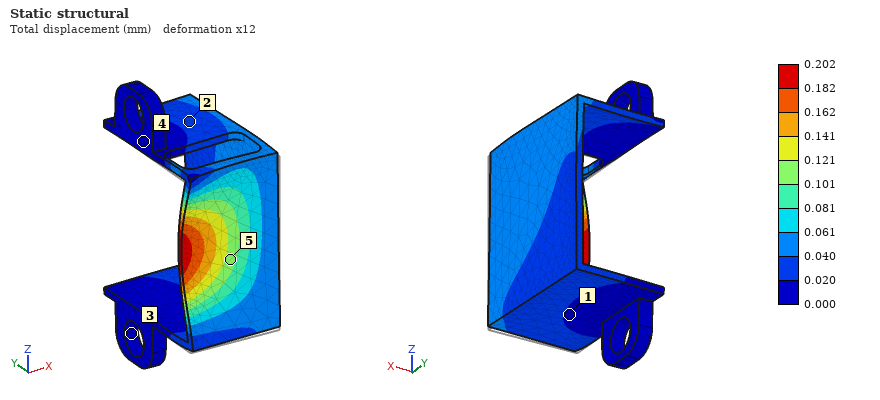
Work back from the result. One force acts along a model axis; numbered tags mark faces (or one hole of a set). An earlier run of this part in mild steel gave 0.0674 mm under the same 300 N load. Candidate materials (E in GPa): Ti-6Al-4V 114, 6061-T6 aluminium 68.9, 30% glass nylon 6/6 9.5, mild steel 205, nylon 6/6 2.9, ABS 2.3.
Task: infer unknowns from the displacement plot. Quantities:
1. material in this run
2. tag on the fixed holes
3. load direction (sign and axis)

6061-T6 aluminium
3
+Y
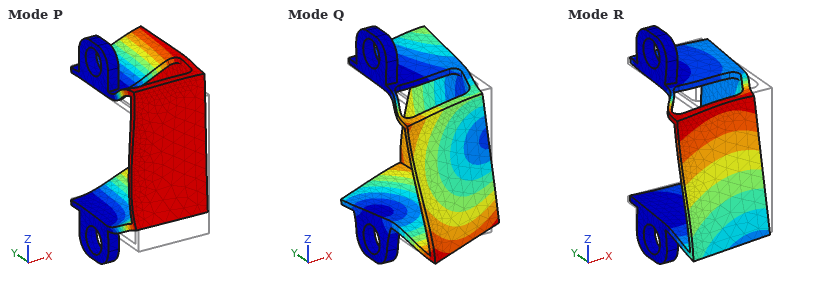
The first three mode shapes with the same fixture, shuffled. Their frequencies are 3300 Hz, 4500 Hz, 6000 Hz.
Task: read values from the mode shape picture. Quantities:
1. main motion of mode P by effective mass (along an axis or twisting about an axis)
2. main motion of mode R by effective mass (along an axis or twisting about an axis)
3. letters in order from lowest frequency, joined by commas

along Z
along X
P, R, Q
